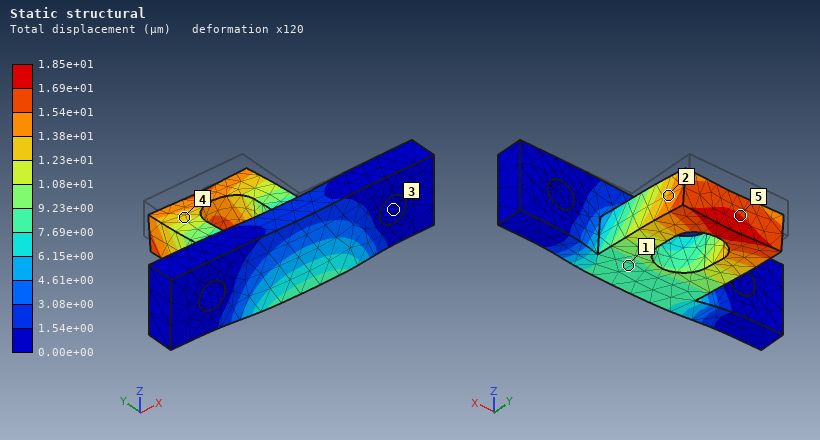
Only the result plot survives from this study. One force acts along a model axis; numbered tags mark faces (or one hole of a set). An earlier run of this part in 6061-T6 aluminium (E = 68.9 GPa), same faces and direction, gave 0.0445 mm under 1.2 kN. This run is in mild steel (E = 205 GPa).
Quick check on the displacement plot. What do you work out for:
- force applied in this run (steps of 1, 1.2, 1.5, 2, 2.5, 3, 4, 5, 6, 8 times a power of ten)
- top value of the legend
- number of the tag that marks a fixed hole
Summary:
1.5 kN
1.85e+01 µm
3
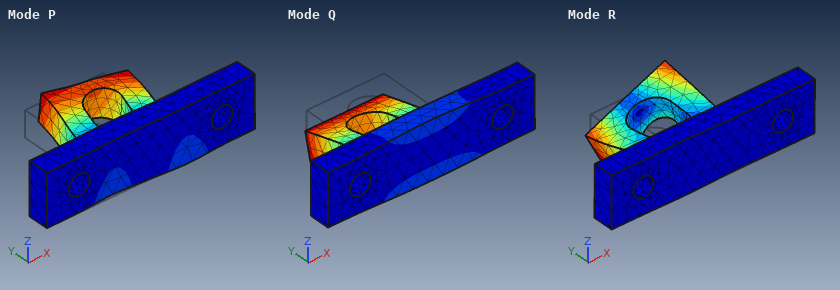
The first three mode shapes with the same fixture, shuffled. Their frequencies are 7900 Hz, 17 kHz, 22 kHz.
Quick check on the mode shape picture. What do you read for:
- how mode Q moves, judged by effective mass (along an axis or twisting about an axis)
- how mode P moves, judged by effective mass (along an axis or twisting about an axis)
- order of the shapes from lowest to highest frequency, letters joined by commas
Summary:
along Z
along X
Q, P, R
